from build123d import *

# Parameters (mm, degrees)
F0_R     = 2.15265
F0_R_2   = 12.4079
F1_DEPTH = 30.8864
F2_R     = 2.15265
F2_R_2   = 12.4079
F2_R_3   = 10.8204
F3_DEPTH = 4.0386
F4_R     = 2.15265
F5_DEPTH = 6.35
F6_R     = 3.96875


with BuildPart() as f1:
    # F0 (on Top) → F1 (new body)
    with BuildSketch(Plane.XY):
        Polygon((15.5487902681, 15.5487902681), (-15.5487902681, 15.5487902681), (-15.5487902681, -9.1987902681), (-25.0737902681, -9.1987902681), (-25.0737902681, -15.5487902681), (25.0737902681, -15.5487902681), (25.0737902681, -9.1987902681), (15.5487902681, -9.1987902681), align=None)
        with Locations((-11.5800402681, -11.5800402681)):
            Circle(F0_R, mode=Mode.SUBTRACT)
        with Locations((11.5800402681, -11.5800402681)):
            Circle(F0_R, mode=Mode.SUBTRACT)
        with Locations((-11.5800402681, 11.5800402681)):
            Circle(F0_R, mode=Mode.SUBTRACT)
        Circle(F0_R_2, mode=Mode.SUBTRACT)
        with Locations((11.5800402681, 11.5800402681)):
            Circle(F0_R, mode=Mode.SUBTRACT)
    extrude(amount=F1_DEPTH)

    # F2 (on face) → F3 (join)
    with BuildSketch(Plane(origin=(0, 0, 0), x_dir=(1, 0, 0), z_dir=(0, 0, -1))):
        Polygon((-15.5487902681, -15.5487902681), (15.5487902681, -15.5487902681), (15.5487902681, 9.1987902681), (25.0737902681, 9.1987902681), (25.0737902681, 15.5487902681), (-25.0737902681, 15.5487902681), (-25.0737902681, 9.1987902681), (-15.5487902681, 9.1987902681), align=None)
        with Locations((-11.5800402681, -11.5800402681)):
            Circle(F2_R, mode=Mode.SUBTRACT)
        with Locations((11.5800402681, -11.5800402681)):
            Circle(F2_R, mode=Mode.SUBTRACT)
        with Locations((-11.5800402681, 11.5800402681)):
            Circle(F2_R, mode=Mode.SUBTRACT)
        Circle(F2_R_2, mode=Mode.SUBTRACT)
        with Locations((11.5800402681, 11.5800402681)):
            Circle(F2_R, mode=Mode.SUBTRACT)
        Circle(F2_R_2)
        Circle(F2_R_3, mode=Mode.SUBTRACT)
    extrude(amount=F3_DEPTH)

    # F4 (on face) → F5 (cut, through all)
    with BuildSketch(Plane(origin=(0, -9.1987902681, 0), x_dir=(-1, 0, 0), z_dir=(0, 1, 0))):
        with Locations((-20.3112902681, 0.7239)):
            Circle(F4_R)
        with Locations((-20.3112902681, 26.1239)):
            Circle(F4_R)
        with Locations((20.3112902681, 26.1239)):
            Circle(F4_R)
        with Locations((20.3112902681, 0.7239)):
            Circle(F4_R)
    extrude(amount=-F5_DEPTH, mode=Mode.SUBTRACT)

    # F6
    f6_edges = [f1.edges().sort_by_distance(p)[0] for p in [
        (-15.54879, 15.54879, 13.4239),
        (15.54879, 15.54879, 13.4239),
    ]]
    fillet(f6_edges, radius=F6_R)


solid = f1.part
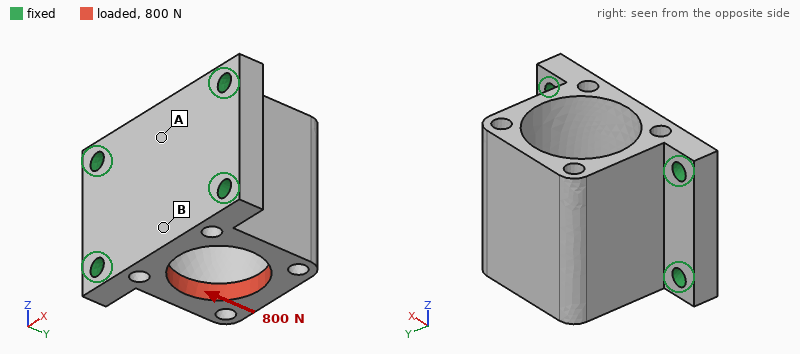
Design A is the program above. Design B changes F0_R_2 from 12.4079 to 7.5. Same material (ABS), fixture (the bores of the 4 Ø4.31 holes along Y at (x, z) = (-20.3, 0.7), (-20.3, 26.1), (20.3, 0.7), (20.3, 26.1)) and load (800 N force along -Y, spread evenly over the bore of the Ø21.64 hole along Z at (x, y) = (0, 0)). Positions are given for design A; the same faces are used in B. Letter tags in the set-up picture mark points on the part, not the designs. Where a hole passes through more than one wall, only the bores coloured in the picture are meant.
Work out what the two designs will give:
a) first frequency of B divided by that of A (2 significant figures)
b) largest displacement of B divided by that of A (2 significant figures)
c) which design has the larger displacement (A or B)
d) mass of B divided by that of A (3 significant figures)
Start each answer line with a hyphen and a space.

- 1.3
- 0.77
- A
- 1.50
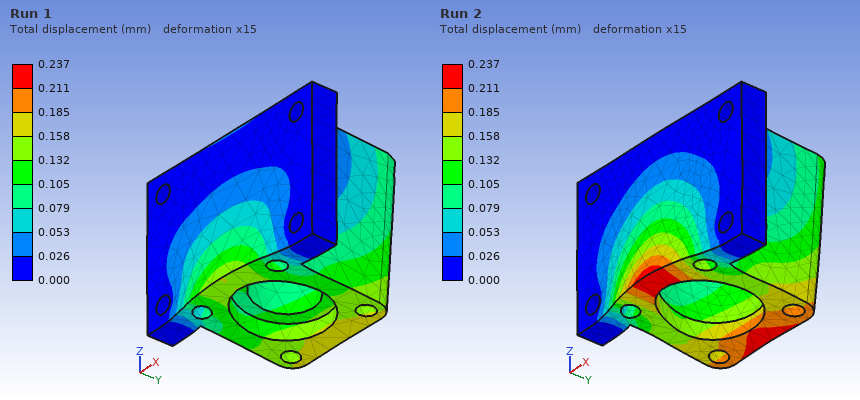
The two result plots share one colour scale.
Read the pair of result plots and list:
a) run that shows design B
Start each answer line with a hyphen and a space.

- Run 1
